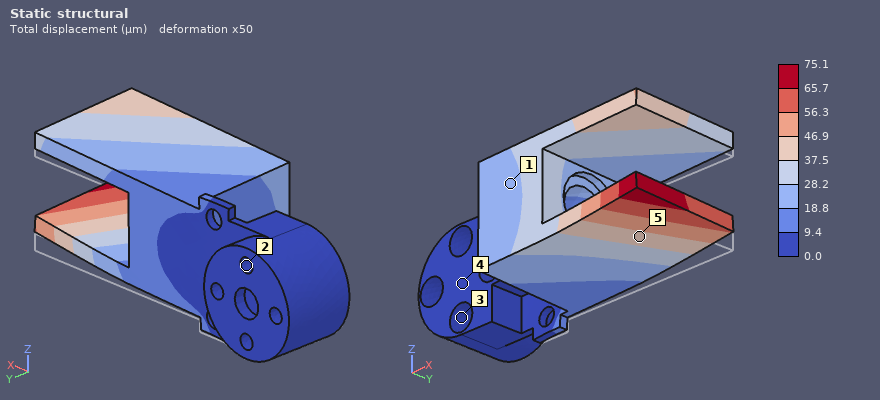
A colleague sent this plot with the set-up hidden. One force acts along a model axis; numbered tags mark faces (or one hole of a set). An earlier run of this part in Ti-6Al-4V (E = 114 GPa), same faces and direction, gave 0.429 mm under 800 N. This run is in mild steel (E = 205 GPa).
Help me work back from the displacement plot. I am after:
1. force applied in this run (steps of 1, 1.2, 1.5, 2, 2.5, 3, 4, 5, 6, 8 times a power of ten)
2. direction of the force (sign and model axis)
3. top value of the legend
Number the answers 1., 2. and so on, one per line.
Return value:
1. 250 N
2. +Z
3. 75.1 µm
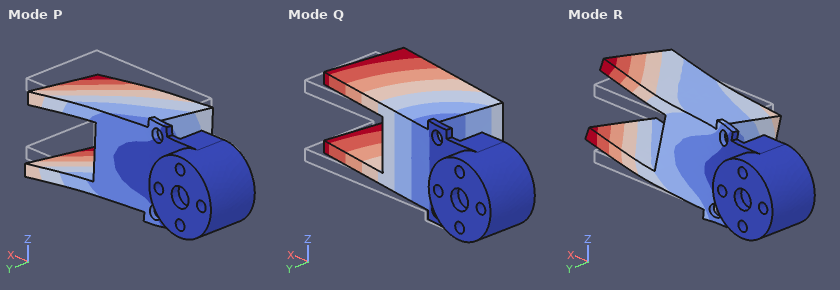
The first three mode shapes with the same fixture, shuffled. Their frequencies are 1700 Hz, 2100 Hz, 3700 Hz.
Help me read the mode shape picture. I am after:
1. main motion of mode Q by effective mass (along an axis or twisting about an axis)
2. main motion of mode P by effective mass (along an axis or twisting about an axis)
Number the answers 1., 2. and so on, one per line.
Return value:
1. along Y
2. along Z
